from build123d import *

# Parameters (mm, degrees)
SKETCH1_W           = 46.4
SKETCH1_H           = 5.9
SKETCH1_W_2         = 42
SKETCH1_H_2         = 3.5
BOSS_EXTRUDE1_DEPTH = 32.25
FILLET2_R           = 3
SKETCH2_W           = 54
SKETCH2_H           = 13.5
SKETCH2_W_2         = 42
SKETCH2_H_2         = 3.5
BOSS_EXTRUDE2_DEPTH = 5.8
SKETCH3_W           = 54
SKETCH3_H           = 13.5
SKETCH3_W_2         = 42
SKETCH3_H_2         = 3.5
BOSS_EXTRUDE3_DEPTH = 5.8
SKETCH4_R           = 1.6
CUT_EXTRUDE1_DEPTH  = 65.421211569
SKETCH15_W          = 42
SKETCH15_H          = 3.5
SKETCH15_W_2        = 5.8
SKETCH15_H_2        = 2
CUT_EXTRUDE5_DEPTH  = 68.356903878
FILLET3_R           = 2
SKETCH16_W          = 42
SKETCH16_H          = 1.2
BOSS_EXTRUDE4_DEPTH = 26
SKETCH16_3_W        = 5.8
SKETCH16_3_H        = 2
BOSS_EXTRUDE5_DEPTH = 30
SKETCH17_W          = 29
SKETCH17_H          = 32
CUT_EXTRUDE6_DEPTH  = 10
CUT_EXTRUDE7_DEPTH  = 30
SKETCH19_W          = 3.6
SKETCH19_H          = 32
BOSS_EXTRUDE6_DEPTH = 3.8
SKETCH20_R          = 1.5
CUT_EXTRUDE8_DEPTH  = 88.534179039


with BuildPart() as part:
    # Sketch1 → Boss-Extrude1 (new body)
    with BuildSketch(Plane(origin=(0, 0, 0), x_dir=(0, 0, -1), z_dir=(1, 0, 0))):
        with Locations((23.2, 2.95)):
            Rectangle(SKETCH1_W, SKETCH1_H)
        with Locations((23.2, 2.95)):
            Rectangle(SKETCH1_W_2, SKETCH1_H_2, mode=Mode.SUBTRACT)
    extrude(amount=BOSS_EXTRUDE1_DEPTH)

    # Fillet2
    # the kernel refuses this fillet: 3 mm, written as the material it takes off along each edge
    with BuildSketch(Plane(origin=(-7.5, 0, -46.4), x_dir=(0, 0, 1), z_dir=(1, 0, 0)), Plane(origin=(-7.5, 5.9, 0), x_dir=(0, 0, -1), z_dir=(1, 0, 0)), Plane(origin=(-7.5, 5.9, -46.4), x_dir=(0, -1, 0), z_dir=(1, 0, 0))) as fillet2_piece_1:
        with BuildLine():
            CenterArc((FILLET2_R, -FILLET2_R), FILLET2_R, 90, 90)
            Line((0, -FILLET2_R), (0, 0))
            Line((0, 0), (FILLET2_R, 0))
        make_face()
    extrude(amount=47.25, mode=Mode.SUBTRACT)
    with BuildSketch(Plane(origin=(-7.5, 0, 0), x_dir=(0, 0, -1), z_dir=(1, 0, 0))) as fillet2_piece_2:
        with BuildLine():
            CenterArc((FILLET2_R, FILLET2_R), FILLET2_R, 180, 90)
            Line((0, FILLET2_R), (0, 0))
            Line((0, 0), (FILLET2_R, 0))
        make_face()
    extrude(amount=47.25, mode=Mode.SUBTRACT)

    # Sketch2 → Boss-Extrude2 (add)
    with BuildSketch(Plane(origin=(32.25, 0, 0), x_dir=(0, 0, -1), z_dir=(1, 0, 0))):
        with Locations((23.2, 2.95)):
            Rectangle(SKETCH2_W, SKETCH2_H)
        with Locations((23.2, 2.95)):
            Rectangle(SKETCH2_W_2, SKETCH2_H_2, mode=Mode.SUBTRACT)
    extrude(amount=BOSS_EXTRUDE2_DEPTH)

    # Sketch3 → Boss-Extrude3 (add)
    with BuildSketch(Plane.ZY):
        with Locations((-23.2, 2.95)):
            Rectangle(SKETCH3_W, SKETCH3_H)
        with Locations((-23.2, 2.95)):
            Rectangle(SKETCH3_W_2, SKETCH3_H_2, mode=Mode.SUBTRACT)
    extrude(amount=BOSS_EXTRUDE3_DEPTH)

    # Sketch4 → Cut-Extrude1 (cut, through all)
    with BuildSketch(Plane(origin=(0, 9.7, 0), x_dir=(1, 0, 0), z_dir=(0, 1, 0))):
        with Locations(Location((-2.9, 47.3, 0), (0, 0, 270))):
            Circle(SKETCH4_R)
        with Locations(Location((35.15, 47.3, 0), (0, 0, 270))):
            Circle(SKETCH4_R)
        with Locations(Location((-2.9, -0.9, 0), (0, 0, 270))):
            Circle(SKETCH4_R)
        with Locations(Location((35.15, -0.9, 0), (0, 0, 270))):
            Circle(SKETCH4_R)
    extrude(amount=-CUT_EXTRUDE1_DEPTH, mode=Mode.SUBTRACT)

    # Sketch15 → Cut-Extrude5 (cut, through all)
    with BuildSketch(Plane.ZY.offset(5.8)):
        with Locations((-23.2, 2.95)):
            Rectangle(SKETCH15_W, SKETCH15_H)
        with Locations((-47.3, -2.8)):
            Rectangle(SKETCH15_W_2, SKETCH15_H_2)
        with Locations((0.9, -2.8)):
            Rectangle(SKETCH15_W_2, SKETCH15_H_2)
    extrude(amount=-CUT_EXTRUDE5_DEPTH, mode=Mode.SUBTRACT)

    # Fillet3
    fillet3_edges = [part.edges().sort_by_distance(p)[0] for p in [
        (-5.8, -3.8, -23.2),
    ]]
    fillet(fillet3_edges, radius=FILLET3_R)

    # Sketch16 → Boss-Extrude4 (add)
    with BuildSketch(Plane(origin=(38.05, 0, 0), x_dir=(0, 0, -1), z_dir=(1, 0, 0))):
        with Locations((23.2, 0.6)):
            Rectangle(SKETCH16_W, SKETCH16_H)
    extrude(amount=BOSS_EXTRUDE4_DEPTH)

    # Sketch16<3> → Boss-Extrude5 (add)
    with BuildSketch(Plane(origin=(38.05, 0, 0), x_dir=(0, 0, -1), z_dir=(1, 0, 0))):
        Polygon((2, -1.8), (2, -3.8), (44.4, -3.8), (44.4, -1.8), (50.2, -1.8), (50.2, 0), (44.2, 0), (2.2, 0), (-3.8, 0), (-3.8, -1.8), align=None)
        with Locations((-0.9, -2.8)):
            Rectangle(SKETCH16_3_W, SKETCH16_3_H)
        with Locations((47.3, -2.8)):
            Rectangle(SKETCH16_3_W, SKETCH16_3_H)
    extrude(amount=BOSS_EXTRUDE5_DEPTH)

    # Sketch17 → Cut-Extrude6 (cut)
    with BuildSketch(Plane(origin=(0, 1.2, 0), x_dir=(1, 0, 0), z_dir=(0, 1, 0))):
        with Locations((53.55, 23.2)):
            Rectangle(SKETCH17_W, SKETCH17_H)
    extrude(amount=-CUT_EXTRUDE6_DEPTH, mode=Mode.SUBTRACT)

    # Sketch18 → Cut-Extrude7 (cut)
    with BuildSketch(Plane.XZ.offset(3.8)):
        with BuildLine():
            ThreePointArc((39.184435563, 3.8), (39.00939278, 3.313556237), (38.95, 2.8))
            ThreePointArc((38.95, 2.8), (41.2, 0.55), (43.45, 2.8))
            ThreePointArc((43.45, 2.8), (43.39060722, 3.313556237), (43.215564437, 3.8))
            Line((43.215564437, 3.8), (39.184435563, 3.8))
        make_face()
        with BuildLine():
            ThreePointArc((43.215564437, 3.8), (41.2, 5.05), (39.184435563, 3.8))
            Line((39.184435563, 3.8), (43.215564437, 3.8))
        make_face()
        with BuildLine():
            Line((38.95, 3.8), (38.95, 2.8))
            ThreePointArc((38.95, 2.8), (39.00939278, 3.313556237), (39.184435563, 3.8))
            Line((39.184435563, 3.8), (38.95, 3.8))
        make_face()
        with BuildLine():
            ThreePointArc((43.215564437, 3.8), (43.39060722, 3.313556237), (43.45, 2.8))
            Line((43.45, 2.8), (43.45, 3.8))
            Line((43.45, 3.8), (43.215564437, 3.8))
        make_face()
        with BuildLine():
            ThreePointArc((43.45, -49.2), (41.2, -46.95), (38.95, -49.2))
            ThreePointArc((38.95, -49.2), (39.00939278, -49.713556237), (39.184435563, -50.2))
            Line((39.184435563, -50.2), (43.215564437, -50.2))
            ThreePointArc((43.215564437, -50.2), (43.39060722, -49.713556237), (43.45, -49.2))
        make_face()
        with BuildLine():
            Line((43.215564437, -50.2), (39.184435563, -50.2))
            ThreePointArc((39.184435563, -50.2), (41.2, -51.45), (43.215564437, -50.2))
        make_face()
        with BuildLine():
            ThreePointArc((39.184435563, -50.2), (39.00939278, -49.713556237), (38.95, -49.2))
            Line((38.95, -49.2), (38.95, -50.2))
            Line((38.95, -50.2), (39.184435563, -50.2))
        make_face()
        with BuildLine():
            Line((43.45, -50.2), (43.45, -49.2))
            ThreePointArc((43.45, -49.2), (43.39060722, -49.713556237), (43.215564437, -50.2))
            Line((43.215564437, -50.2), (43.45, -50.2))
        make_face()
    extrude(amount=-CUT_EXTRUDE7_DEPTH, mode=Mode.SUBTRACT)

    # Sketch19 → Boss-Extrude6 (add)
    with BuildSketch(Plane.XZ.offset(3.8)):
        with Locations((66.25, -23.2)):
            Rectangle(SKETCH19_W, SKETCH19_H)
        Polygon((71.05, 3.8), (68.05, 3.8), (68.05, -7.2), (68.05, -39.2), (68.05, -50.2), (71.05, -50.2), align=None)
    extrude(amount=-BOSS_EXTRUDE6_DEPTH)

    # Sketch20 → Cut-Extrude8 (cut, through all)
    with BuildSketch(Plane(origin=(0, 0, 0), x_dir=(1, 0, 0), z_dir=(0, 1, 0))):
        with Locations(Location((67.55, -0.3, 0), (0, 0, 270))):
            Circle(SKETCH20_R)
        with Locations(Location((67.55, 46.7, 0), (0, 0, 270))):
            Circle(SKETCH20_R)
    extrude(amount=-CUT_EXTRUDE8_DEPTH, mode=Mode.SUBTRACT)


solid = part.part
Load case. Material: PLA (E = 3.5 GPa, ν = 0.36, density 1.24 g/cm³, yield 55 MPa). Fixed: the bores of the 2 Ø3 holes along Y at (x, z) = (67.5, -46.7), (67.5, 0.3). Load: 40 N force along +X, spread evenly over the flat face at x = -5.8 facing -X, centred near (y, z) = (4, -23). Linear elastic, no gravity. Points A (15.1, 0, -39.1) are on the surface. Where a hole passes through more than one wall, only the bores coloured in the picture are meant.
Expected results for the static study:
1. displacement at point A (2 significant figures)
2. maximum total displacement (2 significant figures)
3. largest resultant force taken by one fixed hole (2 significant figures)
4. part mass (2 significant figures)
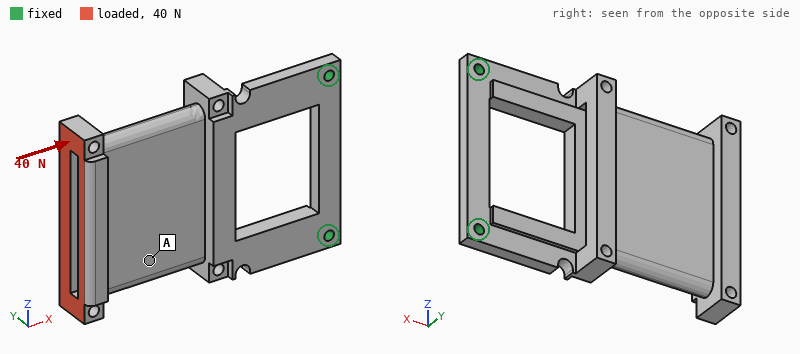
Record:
0.64 mm
1.1 mm
20 N
17 g
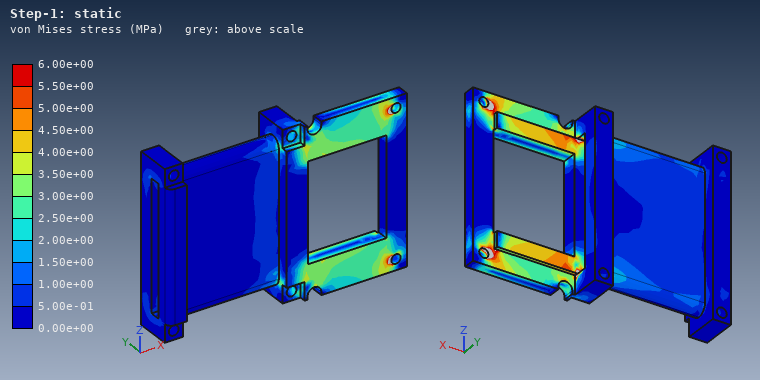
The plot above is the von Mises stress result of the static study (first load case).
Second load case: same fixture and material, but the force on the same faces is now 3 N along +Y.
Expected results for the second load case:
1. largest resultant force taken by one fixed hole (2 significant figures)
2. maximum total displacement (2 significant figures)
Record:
1.7 N
0.86 mm
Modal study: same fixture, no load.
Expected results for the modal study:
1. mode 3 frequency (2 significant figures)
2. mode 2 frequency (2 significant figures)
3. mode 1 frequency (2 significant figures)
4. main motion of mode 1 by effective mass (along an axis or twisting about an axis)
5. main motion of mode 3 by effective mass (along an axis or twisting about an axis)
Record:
760 Hz
560 Hz
130 Hz
along Y
along Y
